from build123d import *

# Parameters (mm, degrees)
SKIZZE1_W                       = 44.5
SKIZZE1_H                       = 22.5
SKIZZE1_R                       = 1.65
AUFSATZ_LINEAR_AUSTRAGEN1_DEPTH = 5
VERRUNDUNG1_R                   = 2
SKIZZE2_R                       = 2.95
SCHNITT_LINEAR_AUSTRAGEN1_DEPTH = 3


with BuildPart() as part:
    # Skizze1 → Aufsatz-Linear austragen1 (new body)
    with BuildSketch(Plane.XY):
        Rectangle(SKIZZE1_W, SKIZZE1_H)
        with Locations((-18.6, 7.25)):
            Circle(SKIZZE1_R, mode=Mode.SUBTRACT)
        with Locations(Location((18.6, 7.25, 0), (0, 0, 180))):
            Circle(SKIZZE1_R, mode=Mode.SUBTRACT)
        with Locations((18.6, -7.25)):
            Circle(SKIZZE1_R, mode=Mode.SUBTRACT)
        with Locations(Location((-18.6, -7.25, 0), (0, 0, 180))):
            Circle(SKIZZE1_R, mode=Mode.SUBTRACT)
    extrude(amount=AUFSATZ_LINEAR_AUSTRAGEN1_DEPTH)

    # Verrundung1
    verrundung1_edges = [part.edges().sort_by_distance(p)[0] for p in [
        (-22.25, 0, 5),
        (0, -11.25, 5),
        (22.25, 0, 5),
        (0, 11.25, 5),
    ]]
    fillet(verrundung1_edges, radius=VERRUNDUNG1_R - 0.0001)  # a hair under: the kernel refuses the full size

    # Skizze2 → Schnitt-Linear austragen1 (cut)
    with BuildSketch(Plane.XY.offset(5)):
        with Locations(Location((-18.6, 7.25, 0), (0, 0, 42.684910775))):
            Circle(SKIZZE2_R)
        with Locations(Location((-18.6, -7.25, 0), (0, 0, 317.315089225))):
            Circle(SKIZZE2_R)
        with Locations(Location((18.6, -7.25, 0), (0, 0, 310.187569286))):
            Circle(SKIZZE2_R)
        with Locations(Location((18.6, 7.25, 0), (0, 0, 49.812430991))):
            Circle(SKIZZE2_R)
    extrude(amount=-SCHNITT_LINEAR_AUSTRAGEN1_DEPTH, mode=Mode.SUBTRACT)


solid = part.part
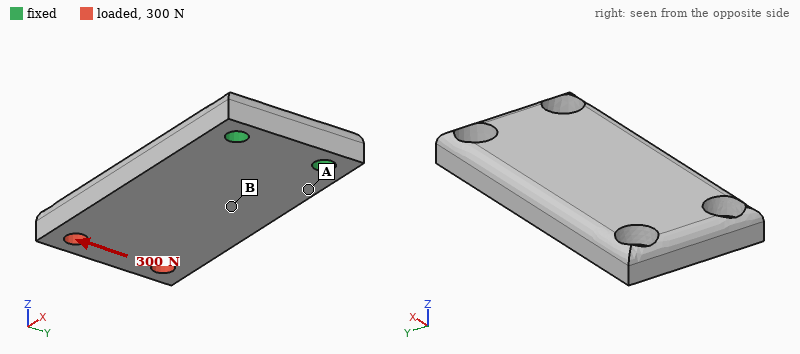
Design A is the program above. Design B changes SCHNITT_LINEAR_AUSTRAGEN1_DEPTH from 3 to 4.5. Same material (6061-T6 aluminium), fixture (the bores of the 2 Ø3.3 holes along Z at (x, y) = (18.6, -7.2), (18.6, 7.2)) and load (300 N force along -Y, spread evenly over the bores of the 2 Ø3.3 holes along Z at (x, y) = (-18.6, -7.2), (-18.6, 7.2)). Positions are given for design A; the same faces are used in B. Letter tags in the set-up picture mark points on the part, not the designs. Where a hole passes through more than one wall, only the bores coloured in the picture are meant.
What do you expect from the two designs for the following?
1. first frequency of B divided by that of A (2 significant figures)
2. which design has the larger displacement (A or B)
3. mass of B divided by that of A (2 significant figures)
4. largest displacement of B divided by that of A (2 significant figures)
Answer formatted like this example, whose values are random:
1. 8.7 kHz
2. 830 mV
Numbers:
1. 0.46
2. B
3. 0.97
4. 1.9
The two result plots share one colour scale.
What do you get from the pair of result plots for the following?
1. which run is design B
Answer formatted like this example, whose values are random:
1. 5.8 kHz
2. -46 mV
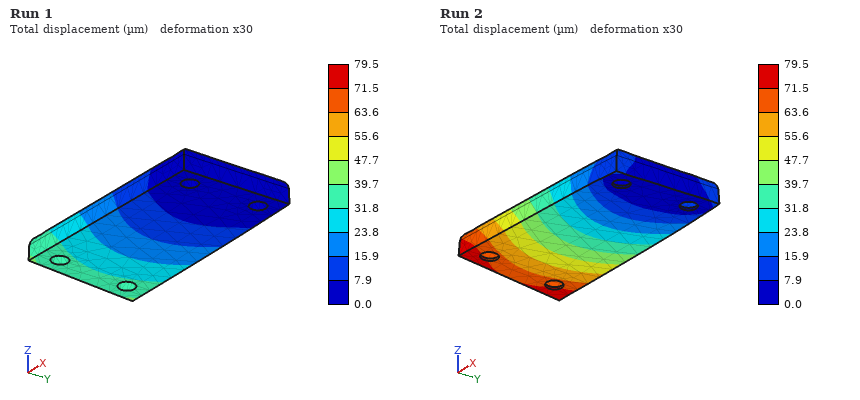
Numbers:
1. Run 2
